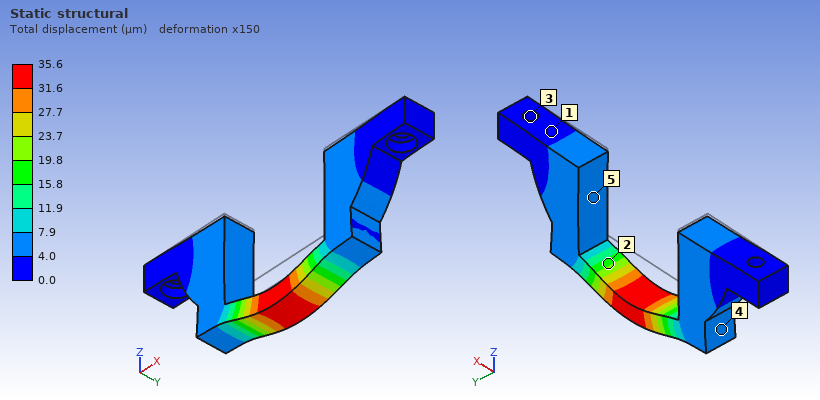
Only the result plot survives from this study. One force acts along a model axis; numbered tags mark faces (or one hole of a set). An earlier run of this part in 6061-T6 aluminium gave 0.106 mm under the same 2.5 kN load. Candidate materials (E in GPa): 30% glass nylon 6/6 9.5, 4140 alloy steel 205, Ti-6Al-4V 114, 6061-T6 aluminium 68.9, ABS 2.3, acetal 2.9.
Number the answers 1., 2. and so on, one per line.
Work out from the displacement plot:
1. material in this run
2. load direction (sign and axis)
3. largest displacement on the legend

1. 4140 alloy steel
2. -Z
3. 35.6 µm
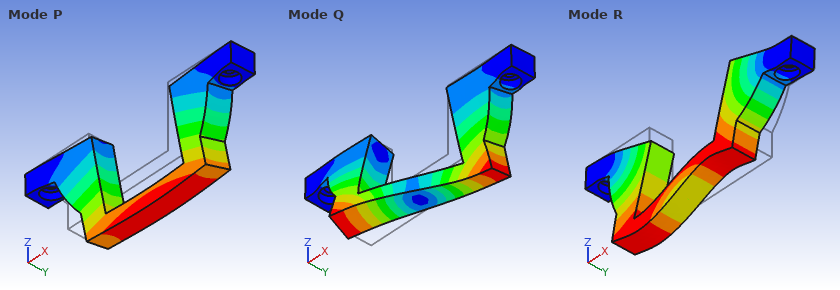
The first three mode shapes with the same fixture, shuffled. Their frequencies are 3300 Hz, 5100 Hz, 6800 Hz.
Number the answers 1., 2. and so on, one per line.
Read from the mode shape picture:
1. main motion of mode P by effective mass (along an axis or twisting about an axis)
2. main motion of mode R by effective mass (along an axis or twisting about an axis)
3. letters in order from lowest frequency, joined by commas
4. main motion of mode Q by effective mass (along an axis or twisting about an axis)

1. along Y
2. along X
3. P, R, Q
4. twisting about Z
